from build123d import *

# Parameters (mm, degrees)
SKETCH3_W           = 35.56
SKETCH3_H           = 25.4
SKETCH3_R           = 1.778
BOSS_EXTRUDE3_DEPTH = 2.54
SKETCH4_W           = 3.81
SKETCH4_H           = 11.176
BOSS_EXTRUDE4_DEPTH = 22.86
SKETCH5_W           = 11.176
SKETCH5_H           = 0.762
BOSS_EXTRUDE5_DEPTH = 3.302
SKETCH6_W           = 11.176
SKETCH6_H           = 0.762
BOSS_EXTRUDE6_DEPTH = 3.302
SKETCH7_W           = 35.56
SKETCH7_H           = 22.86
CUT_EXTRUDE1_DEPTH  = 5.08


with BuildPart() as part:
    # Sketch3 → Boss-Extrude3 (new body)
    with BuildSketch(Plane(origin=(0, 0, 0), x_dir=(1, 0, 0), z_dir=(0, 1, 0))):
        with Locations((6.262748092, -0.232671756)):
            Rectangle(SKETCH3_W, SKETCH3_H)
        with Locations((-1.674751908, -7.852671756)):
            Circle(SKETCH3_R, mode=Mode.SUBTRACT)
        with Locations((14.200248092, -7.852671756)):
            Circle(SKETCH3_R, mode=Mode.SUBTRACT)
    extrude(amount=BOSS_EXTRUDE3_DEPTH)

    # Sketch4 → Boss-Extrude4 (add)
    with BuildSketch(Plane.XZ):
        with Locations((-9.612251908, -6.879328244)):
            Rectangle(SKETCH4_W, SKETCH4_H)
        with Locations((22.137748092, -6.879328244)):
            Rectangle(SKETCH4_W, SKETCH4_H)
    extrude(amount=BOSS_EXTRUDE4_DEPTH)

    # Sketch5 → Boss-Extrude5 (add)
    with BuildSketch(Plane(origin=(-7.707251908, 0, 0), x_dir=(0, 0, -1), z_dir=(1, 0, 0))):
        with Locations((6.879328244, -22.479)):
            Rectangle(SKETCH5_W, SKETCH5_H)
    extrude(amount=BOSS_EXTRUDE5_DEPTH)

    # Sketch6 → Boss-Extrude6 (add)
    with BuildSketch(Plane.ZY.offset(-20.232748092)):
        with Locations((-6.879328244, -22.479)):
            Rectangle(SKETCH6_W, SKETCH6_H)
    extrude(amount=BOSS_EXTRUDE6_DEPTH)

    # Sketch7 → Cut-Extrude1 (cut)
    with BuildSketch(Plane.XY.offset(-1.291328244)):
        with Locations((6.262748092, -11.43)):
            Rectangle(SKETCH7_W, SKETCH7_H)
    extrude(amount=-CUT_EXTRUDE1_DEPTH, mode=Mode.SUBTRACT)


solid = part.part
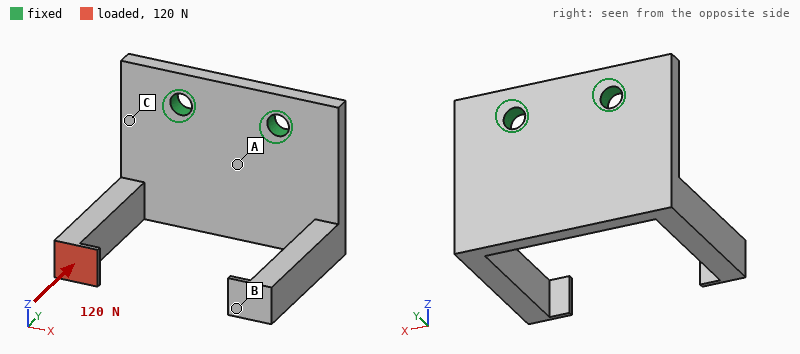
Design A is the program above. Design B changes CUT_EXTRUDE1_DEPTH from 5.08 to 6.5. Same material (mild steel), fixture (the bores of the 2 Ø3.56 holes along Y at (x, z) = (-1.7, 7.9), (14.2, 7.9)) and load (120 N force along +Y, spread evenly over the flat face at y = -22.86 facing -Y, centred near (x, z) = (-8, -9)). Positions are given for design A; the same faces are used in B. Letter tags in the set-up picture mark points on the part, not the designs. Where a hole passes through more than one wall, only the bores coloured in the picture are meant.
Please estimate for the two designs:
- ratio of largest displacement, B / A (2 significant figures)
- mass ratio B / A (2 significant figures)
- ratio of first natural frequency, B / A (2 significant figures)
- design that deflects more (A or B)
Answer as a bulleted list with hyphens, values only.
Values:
- 1.1
- 0.92
- 1.1
- B
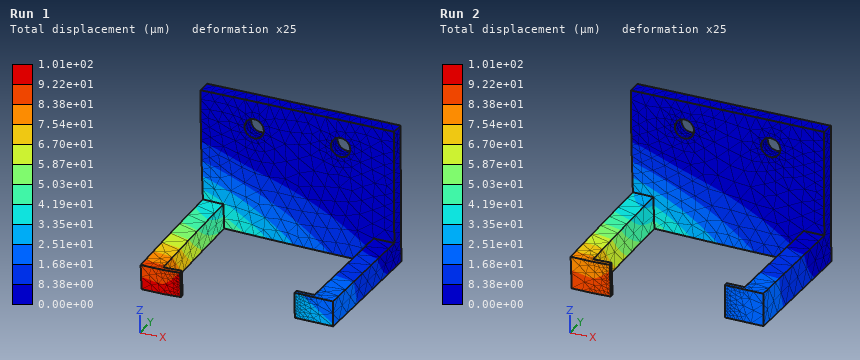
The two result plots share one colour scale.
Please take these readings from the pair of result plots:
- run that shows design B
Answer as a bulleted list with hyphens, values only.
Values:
- Run 1
